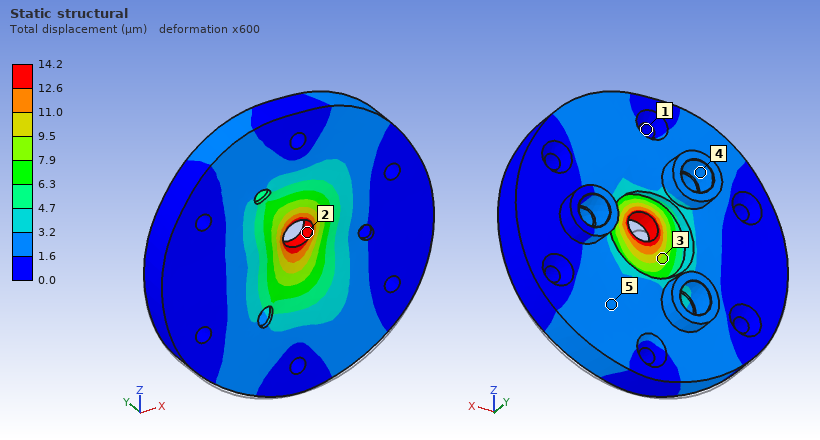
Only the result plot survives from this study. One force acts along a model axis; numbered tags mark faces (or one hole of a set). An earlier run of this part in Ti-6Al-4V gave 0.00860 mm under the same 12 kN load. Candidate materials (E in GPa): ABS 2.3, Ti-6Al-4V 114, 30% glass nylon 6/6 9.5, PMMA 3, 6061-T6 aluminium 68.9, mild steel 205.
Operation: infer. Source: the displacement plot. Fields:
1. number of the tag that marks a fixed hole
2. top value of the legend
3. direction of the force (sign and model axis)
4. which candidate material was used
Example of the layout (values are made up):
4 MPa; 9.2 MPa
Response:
1; 14.2 µm; +Z; 6061-T6 aluminium
